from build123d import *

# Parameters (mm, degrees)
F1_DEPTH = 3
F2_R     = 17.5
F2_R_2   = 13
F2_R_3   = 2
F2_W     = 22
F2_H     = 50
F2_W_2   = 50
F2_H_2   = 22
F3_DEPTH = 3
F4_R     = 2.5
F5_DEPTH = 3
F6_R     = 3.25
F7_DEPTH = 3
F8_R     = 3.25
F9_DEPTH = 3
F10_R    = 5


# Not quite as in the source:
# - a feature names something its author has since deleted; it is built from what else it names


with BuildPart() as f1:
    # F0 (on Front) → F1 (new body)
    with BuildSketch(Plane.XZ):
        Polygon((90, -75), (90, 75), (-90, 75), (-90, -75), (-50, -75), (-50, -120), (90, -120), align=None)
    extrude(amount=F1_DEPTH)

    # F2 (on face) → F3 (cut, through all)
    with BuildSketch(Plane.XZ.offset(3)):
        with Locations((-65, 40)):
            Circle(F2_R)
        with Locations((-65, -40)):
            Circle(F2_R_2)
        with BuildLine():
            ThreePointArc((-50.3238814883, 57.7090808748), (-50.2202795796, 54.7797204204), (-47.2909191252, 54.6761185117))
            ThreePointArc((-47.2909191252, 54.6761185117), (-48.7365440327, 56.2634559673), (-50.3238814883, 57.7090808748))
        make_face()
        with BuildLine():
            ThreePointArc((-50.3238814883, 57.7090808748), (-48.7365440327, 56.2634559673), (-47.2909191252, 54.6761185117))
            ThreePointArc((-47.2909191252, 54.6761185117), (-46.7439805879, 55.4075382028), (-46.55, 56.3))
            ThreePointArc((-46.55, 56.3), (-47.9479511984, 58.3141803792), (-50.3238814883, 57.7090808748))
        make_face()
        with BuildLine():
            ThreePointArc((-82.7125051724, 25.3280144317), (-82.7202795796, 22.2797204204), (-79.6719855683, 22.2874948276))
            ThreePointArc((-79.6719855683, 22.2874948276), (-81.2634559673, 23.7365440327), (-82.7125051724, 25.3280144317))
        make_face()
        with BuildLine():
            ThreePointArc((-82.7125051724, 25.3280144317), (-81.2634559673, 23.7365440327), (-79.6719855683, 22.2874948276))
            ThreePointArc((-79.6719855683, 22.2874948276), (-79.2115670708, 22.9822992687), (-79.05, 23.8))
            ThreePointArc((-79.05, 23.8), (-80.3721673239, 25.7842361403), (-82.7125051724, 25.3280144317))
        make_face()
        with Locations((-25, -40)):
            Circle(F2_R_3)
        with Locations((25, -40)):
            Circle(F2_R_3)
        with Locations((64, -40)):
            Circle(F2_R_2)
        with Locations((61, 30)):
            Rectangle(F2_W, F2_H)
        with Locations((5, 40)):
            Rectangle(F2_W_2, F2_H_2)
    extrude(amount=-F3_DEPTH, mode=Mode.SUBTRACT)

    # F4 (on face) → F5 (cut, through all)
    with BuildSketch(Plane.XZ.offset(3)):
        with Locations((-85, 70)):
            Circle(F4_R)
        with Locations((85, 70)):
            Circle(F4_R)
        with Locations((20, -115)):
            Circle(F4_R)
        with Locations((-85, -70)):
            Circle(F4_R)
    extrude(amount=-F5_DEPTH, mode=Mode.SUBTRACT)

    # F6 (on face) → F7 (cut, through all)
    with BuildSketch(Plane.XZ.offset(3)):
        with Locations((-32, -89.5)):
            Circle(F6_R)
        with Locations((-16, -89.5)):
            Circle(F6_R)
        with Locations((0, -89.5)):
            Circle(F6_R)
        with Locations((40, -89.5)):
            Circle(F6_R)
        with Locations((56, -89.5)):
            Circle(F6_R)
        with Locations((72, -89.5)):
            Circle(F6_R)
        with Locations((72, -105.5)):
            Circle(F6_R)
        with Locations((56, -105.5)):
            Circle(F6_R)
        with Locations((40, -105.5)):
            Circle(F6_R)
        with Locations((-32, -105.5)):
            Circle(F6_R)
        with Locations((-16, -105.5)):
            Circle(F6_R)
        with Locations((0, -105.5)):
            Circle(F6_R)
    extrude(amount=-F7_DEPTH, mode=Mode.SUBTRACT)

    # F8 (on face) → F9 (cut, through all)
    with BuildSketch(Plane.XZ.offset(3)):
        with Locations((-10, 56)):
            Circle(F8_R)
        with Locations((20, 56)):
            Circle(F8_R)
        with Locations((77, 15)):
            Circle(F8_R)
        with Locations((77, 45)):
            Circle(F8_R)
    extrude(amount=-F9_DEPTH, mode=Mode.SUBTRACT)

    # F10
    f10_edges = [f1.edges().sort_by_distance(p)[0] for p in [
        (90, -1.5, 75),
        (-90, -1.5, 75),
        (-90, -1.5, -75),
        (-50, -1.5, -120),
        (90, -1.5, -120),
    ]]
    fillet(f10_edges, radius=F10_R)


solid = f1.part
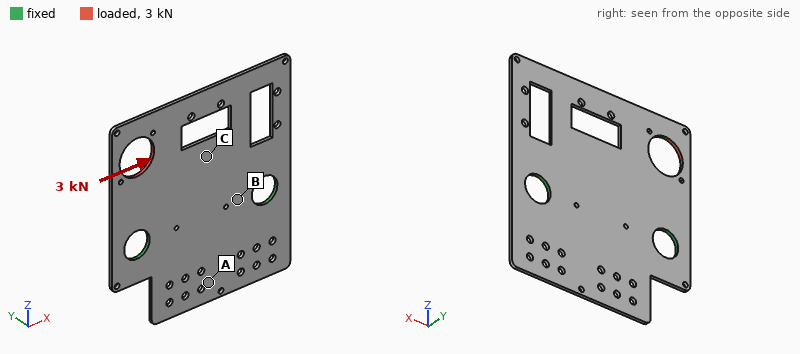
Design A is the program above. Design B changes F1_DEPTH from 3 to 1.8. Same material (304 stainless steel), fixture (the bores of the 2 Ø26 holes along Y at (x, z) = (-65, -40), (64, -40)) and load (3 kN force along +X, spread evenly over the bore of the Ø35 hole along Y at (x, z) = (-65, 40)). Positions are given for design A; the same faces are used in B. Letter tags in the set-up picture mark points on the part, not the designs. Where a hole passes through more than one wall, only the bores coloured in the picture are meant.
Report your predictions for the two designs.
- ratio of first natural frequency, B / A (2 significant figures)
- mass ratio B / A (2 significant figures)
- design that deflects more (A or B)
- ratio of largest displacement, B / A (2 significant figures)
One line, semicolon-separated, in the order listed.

0.60; 0.60; B; 1.7
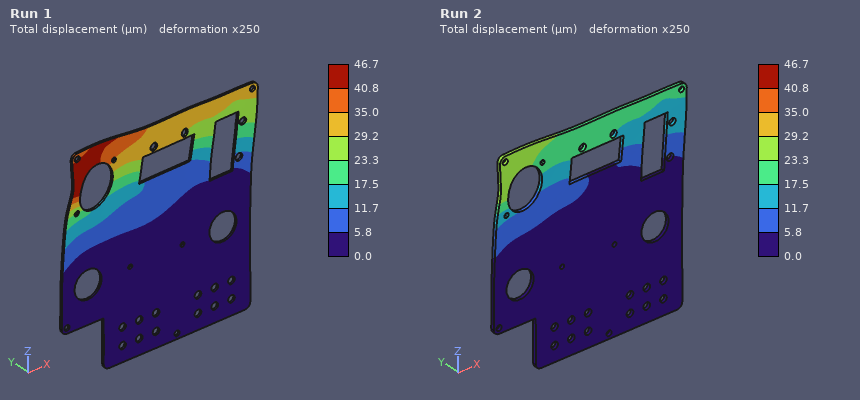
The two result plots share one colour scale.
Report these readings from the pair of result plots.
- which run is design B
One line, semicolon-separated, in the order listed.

Run 1
